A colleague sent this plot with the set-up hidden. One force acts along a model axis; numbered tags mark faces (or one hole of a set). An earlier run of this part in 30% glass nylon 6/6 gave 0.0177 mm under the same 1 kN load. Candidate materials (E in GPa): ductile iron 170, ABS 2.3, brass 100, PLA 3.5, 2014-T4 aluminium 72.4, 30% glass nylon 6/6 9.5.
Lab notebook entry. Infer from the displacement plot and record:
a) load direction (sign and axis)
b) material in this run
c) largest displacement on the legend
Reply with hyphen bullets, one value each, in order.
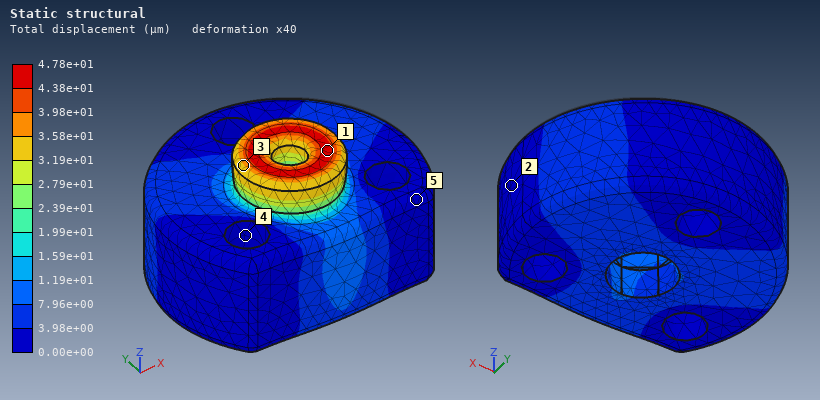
- -Z
- PLA
- 4.78e+01 µm
